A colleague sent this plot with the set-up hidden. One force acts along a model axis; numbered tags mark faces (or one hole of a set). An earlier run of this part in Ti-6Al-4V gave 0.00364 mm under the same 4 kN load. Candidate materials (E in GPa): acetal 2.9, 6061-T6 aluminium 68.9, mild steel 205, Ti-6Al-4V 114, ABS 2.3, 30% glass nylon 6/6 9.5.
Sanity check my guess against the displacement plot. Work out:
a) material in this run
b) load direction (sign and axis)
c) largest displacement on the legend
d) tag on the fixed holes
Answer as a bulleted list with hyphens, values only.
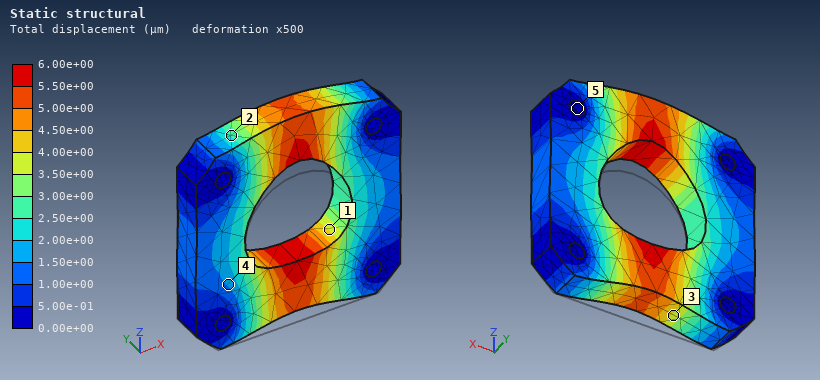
- 6061-T6 aluminium
- +Z
- 6.00e+00 µm
- 5
